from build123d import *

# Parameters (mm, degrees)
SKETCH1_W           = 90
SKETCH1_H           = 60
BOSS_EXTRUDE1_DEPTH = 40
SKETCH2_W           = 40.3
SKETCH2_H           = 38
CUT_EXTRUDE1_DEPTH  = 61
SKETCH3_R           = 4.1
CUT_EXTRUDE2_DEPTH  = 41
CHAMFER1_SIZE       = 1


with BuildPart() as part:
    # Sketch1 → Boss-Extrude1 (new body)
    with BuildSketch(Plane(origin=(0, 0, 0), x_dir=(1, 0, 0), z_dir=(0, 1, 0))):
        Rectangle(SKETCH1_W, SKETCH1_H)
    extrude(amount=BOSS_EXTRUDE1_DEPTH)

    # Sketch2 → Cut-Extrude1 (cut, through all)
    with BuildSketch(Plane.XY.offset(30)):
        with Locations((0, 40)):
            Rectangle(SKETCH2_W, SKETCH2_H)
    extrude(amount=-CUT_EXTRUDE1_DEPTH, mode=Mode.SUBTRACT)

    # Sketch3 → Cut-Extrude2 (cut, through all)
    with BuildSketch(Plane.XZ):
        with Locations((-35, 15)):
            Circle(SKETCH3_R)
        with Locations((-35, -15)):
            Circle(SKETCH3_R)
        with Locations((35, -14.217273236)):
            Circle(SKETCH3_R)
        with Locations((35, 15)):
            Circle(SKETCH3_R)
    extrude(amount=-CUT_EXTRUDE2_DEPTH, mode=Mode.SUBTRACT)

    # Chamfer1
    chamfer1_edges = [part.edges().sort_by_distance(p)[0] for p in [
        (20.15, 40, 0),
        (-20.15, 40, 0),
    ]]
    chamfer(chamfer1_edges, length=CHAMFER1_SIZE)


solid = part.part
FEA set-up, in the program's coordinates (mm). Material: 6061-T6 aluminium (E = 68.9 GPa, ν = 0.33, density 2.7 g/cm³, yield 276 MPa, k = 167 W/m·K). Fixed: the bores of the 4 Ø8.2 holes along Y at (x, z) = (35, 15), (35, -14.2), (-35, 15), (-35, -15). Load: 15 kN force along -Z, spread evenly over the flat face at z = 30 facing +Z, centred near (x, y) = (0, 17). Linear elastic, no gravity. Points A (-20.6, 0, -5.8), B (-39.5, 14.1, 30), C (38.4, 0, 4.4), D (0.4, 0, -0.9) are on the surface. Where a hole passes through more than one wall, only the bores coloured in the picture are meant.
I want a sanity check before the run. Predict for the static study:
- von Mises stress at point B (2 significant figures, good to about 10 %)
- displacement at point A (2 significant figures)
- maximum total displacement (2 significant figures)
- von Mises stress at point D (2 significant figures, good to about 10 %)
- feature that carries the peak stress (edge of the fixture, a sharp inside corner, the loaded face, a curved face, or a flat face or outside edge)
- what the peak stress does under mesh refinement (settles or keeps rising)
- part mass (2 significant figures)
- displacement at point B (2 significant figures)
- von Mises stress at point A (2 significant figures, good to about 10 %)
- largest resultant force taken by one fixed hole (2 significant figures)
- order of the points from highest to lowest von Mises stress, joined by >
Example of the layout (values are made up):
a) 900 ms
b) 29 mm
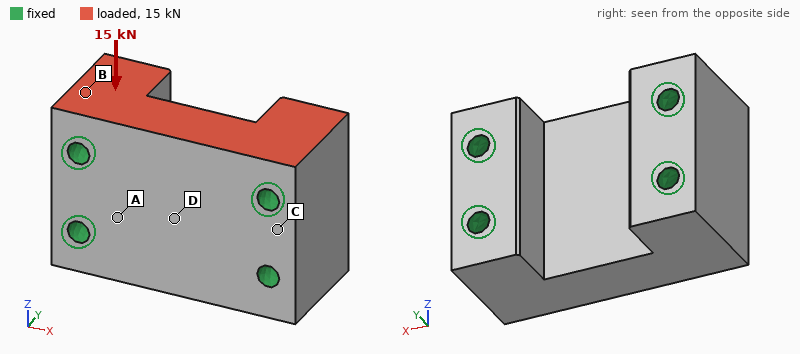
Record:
a) 6.4 MPa
b) 1.2 µm
c) 4.2 µm
d) 2.5 MPa
e) edge of the fixture
f) keeps rising
g) 440 g
h) 1.0 µm
i) 4.5 MPa
j) 5.8 kN
k) B > A > D > C
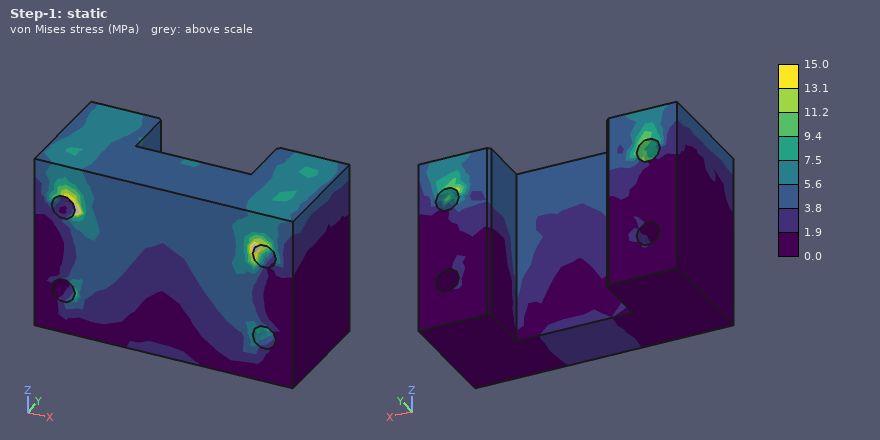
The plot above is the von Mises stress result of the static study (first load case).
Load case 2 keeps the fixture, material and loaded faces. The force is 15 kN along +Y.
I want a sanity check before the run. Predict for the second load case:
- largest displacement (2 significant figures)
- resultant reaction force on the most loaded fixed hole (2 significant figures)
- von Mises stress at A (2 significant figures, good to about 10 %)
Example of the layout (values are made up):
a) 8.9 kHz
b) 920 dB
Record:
a) 15 µm
b) 7.7 kN
c) 5.7 MPa
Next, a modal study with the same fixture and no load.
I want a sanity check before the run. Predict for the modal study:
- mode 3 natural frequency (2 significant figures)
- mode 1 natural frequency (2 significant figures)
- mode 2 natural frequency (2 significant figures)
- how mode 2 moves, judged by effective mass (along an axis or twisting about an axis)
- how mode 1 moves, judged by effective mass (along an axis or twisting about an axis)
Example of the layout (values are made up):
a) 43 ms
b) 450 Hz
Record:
a) 22 kHz
b) 19 kHz
c) 20 kHz
d) along Z
e) along Y
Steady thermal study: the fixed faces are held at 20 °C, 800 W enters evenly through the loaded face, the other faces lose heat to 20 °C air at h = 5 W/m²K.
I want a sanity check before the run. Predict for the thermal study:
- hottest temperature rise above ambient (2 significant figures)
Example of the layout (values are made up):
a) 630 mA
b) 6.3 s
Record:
a) 45 K
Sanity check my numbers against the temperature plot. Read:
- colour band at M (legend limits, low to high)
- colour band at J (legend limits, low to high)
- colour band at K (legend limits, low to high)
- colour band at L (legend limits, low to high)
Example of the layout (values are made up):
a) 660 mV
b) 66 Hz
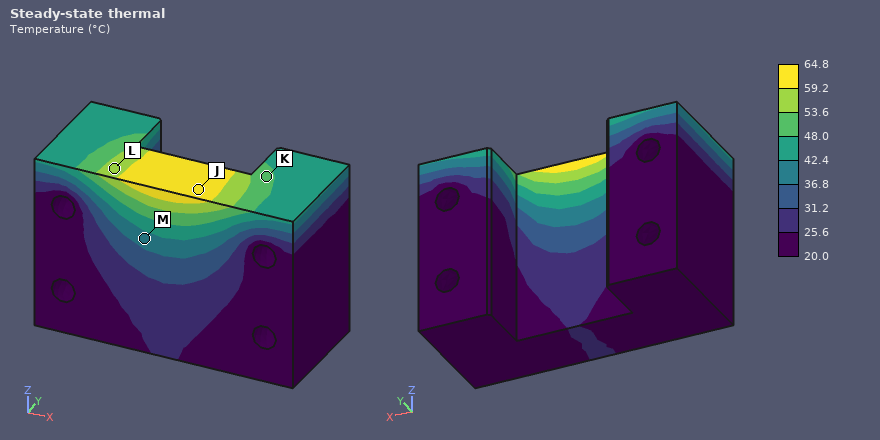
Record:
a) 36.8 to 42.4 °C
b) 59.2 to 64.8 °C
c) 48.0 to 53.6 °C
d) 53.6 to 59.2 °C
